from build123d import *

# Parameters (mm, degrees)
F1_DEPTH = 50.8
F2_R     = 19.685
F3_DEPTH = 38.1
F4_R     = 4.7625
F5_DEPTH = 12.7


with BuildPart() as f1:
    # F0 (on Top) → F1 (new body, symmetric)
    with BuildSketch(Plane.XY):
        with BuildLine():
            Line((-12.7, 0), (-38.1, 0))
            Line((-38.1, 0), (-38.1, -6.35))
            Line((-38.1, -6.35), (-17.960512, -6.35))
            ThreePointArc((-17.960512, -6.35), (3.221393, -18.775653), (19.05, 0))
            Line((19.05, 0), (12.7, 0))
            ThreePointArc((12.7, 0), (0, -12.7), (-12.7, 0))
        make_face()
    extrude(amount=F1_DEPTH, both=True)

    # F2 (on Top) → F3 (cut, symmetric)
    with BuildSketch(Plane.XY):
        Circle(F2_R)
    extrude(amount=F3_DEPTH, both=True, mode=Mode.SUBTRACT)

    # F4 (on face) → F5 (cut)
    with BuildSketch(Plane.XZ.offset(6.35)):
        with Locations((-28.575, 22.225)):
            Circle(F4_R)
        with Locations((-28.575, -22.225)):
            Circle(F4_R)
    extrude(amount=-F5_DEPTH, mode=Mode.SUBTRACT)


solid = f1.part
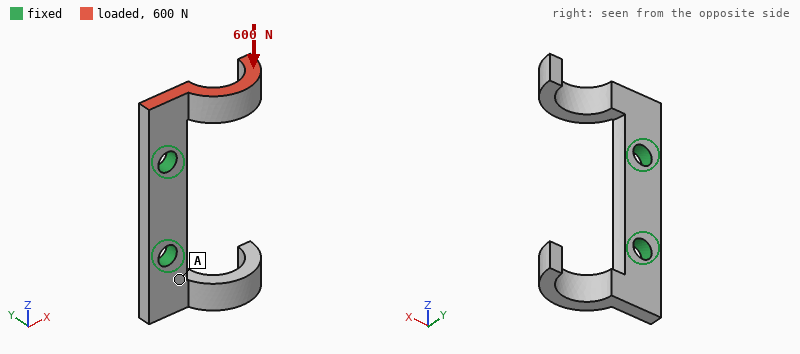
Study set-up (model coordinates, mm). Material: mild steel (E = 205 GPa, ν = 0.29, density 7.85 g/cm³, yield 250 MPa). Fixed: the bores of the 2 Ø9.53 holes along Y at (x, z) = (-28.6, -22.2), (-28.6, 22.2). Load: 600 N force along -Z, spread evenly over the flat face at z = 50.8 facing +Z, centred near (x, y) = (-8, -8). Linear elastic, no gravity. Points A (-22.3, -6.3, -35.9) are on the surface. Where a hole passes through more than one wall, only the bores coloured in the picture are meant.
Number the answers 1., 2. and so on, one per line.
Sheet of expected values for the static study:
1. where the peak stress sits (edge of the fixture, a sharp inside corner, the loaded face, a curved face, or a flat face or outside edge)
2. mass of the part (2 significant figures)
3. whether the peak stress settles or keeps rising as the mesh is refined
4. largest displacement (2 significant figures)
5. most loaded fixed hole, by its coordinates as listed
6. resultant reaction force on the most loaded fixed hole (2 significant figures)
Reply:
1. a sharp inside corner
2. 150 g
3. keeps rising
4. 67 µm
5. (-28.6, 22.2)
6. 600 N
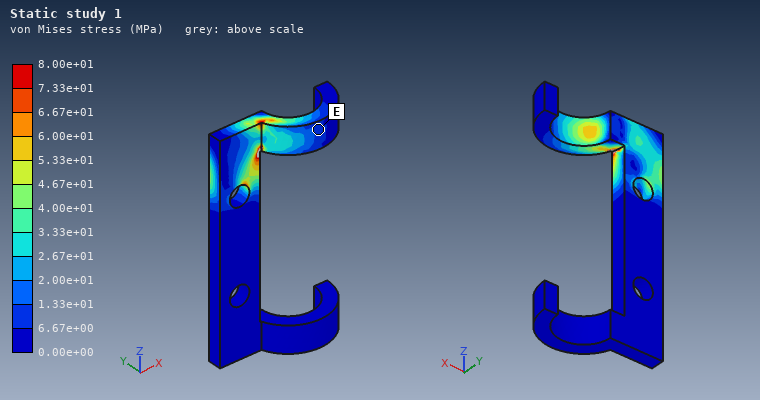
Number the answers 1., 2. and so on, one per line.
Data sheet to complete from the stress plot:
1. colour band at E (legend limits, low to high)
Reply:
1. 6.67e+00 to 1.33e+01 MPa
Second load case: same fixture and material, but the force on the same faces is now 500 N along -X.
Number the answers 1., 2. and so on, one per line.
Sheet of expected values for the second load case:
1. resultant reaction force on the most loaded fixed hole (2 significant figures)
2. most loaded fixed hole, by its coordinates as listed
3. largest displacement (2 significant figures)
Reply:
1. 550 N
2. (-28.6, 22.2)
3. 48 µm
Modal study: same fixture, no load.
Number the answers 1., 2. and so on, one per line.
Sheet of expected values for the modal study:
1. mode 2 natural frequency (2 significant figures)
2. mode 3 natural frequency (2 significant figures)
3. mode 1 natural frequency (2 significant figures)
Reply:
1. 1500 Hz
2. 2700 Hz
3. 1500 Hz
